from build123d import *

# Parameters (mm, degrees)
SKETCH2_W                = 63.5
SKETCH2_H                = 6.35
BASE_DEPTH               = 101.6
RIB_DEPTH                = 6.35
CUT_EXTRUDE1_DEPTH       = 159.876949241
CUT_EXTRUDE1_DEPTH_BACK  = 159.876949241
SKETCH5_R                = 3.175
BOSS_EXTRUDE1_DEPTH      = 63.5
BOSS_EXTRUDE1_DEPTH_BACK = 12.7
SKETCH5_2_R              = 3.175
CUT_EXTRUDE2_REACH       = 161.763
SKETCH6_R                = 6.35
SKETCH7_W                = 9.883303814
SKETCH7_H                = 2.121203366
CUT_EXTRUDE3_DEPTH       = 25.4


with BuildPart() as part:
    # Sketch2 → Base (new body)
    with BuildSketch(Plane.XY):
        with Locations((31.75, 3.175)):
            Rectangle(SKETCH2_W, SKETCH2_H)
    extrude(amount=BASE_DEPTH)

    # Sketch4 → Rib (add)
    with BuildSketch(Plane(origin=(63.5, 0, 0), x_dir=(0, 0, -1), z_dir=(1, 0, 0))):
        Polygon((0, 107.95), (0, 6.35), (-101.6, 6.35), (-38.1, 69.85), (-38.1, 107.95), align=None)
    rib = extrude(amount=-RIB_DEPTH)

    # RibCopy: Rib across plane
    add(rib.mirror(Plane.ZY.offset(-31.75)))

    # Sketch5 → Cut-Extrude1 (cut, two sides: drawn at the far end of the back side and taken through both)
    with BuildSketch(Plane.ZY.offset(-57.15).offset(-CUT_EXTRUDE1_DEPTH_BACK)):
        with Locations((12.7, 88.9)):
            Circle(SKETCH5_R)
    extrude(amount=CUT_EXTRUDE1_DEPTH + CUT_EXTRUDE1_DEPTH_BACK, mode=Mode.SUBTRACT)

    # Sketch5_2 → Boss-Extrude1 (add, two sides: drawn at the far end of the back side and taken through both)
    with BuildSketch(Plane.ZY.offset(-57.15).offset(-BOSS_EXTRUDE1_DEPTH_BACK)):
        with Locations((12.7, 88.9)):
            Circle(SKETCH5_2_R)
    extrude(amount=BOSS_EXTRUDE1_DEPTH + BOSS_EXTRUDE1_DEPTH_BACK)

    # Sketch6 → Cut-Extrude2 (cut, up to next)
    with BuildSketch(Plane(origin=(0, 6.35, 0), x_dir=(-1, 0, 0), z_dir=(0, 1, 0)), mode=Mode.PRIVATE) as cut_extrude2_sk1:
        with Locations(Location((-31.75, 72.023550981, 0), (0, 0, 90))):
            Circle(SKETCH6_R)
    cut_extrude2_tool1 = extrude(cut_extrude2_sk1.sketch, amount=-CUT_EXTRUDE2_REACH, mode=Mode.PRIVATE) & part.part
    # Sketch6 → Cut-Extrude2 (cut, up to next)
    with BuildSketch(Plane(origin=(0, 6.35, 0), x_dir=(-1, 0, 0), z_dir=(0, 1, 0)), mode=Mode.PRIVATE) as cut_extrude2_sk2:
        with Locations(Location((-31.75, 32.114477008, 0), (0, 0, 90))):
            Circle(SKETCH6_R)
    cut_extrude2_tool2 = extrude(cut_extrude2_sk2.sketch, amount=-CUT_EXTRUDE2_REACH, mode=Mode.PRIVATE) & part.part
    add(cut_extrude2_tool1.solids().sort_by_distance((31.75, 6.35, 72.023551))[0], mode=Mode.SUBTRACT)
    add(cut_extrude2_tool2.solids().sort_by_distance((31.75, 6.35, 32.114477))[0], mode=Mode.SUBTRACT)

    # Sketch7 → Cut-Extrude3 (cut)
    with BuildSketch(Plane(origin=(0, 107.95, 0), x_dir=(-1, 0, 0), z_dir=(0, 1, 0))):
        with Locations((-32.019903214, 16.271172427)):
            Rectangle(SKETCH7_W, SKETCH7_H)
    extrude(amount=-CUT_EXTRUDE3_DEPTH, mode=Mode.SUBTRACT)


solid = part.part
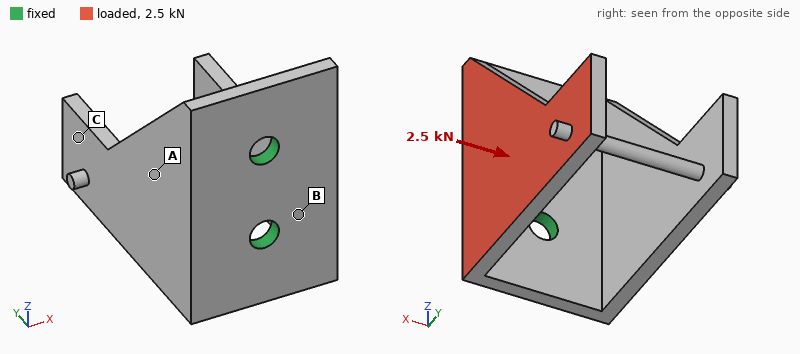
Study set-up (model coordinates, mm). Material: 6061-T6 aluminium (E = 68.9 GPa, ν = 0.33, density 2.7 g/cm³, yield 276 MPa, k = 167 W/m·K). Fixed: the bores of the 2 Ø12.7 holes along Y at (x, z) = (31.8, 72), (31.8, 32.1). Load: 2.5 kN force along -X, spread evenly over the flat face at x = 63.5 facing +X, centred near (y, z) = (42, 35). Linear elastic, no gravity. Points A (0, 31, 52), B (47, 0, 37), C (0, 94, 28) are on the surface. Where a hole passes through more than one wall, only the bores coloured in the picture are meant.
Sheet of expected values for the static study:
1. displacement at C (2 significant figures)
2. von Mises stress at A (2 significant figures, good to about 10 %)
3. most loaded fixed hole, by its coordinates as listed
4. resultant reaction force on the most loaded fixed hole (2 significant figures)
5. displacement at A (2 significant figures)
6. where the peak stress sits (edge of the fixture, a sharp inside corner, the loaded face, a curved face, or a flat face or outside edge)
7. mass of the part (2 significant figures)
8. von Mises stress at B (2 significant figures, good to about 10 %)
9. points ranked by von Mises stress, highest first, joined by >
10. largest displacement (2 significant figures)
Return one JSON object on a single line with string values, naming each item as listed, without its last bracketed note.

{"displacement at C": "1.3 mm", "von Mises stress at A": "45 MPa", "most loaded fixed hole, by its coordinates as listed": "(31.8, 32.1)", "resultant reaction force on the most loaded fixed hole": "2.1 kN", "displacement at A": "0.26 mm", "where the peak stress sits": "a curved face", "mass of the part": "310 g", "von Mises stress at B": "90 MPa", "points ranked by von Mises stress, highest first, joined by >": "B > A > C", "largest displacement": "1.7 mm"}
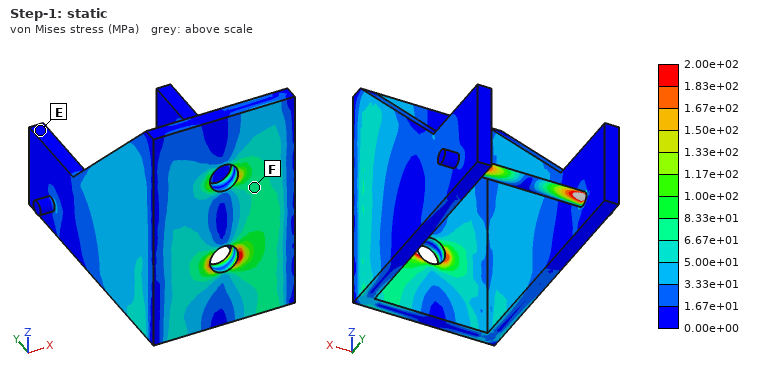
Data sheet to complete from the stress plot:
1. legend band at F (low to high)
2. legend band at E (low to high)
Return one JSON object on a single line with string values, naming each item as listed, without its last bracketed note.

{"legend band at F": "6.67e+01 to 8.33e+01 MPa", "legend band at E": "0.00e+00 to 1.67e+01 MPa"}
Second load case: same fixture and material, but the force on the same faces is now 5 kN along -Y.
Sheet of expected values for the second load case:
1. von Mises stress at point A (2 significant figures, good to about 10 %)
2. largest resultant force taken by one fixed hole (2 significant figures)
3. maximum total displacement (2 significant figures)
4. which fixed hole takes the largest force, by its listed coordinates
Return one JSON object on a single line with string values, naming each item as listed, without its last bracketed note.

{"von Mises stress at point A": "25 MPa", "largest resultant force taken by one fixed hole": "4.1 kN", "maximum total displacement": "1.0 mm", "which fixed hole takes the largest force, by its listed coordinates": "(31.8, 32.1)"}
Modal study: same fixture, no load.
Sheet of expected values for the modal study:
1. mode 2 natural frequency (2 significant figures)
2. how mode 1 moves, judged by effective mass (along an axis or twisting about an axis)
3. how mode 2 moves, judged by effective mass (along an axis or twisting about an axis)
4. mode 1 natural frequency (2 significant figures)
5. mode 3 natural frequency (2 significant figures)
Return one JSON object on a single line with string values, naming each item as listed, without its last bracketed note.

{"mode 2 natural frequency": "1400 Hz", "how mode 1 moves, judged by effective mass": "along X", "how mode 2 moves, judged by effective mass": "along Z", "mode 1 natural frequency": "510 Hz", "mode 3 natural frequency": "1500 Hz"}
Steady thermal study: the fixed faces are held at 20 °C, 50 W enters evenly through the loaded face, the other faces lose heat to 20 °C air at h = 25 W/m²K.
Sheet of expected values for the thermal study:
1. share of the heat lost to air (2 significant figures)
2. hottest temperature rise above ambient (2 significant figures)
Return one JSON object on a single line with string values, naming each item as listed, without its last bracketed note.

{"share of the heat lost to air": "15 %", "hottest temperature rise above ambient": "33 K"}
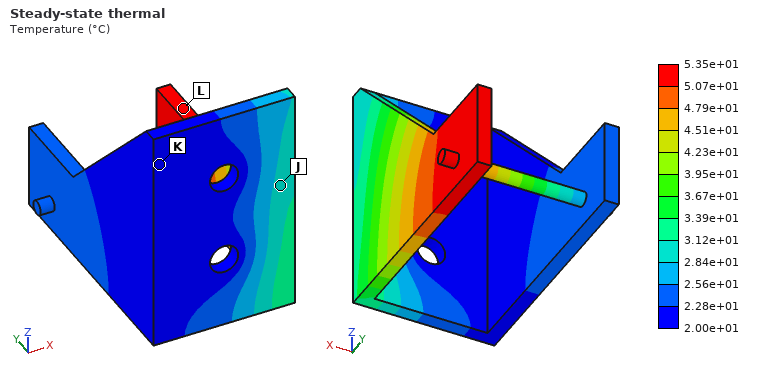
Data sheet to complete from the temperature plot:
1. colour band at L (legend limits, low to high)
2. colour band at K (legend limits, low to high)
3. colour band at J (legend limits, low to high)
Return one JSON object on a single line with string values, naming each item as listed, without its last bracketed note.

{"colour band at L": "5.07e+01 to 5.35e+01 °C", "colour band at K": "2.00e+01 to 2.28e+01 °C", "colour band at J": "2.84e+01 to 3.12e+01 °C"}
